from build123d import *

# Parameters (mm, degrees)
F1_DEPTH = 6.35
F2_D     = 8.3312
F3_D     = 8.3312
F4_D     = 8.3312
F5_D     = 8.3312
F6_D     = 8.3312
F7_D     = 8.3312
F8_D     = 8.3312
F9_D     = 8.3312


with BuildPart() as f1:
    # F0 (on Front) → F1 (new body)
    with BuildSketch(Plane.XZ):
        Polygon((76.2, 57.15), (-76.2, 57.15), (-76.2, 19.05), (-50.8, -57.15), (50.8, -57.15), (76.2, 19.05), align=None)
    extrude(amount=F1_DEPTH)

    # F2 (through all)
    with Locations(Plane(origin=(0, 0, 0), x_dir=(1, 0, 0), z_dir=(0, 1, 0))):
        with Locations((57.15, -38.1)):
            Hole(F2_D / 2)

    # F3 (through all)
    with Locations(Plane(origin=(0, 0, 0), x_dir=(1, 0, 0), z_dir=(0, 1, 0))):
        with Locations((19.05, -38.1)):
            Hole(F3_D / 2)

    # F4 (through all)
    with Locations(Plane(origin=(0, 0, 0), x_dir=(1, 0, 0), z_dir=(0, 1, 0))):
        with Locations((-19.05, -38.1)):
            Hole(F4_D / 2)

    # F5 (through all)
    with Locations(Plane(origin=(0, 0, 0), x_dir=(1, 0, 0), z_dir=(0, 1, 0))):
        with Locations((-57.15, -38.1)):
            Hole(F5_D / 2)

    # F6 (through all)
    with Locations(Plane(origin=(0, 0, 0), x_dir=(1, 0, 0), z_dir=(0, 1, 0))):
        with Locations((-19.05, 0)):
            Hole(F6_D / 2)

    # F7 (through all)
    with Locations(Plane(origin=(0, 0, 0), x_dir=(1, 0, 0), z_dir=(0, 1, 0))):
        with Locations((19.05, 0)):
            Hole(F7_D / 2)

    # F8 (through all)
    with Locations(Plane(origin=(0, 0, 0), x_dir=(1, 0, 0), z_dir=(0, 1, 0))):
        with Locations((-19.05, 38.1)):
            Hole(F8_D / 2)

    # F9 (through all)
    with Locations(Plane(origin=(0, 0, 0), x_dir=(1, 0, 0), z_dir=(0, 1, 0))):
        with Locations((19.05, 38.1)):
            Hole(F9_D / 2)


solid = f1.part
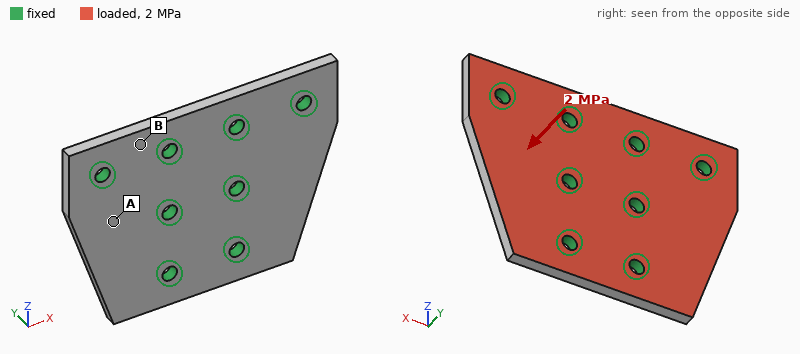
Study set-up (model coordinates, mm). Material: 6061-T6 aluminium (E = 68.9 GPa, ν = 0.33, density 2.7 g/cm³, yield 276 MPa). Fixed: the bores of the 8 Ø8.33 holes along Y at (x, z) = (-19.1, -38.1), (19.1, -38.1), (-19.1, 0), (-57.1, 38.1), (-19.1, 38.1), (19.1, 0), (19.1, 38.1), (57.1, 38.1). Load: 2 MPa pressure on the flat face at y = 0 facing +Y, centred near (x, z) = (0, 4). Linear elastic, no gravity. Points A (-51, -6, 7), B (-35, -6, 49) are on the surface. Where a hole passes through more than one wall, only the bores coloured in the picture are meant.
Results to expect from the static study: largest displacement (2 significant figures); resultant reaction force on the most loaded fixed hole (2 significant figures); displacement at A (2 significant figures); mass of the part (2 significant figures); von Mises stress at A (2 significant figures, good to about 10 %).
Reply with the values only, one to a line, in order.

0.34 mm
4.5 kN
0.13 mm
260 g
60 MPa
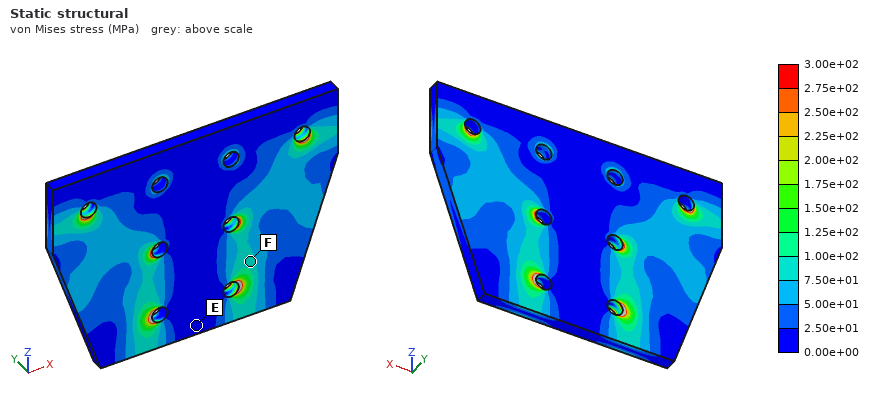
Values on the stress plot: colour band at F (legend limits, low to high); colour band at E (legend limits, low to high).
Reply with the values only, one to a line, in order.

7.50e+01 to 1.00e+02 MPa
0.00e+00 to 2.50e+01 MPa
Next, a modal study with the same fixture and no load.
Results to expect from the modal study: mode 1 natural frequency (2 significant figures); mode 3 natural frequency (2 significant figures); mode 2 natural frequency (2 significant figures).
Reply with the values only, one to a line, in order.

3900 Hz
6700 Hz
3900 Hz
